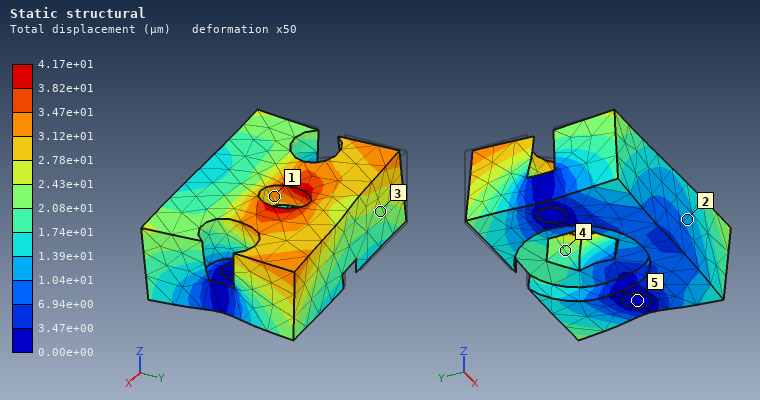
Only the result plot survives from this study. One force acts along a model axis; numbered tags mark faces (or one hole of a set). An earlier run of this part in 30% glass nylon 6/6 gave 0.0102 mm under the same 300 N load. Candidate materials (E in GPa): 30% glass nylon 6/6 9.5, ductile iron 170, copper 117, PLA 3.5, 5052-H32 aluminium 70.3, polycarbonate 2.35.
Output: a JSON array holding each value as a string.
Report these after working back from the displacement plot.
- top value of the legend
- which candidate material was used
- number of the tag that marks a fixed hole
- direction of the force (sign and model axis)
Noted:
["4.17e+01 µm", "polycarbonate", "5", "+X"]
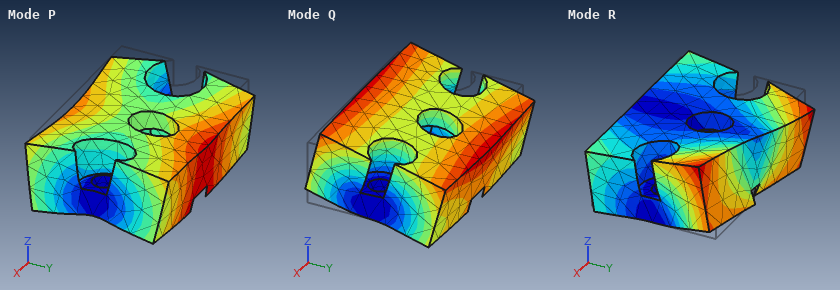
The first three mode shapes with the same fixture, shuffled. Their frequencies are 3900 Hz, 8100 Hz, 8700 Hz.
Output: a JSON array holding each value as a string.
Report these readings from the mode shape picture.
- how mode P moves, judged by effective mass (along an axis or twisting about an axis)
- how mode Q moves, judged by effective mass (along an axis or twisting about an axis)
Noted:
["along Z", "along Y"]
